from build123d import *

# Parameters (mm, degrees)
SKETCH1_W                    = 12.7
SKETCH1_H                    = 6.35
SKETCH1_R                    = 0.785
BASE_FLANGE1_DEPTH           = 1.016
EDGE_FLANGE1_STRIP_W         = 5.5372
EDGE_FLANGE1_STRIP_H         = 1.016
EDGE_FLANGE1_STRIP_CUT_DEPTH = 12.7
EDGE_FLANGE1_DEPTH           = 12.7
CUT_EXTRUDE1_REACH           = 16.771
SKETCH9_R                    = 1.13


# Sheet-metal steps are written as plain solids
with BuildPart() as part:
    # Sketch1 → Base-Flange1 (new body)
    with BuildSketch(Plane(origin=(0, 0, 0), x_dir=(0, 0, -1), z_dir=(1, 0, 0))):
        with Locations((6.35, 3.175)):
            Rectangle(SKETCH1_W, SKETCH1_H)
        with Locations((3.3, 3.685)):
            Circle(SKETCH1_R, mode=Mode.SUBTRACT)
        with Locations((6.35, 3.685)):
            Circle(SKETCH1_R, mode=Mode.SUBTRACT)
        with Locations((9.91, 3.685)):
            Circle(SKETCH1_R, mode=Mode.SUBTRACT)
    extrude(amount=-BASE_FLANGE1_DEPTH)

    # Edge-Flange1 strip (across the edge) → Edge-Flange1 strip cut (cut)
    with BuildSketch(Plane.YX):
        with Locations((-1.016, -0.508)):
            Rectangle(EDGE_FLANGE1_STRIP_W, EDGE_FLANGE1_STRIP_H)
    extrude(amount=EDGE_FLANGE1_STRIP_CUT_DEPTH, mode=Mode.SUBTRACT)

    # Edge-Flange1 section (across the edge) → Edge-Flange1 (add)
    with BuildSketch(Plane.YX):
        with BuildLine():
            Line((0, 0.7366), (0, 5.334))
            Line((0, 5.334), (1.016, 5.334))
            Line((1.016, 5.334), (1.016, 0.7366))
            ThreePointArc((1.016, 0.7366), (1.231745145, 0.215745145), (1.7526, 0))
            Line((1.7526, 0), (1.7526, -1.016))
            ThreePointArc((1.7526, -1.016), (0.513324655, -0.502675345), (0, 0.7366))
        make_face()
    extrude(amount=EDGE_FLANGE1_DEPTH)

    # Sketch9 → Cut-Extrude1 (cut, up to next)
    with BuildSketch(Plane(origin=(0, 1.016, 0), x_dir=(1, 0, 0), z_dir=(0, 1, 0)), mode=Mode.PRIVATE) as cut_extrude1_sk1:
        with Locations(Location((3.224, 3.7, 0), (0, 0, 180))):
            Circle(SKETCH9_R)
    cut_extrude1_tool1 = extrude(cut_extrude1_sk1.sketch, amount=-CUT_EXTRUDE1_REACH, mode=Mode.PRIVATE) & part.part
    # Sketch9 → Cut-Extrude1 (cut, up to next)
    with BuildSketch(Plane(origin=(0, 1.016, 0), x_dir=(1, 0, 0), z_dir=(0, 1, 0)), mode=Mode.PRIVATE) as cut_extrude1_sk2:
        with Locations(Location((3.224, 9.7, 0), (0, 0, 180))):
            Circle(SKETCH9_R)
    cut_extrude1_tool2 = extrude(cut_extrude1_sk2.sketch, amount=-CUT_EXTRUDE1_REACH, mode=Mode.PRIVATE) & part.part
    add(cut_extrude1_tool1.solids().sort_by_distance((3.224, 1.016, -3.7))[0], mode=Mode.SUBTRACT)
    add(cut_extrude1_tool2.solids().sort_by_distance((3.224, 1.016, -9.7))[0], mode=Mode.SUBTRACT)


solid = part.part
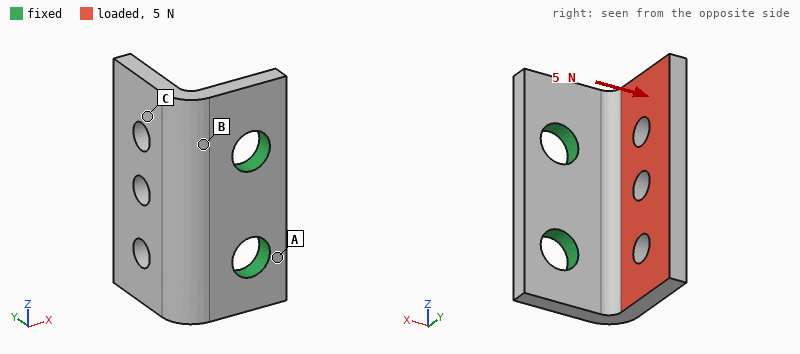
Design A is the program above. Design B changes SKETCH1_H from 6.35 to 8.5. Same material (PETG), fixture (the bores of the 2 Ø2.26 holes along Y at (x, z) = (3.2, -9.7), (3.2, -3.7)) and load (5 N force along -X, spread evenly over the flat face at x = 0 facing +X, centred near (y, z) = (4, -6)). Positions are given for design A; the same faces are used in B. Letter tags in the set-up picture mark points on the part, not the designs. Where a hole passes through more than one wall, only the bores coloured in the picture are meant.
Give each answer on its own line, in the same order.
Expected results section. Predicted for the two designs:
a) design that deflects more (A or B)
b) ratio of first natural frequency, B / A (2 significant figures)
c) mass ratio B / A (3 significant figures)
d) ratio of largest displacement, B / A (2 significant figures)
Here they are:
B
0.76
1.11
1.5
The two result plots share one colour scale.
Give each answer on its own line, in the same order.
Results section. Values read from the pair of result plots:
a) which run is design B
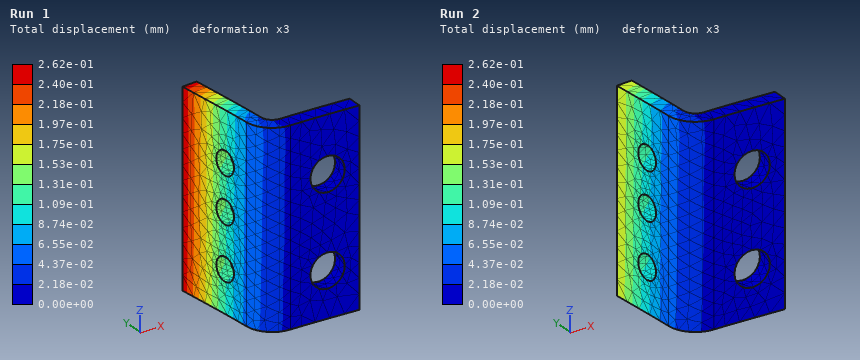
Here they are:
Run 1
